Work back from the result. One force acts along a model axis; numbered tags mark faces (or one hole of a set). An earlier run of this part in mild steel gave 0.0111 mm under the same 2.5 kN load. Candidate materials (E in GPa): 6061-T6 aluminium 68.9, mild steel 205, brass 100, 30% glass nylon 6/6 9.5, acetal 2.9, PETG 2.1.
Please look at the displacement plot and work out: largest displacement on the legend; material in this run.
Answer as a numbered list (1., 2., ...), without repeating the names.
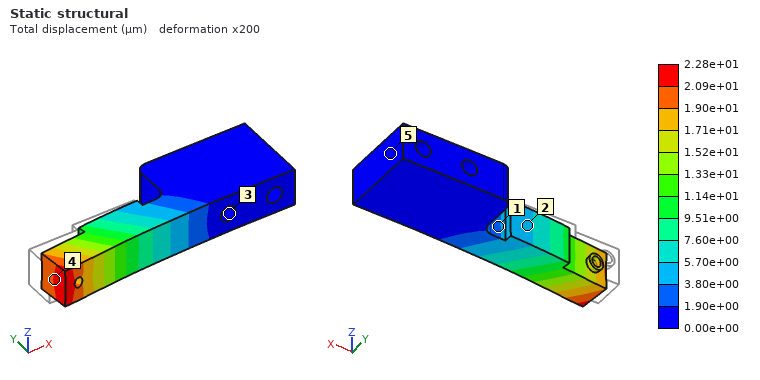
1. 2.28e+01 µm
2. brass
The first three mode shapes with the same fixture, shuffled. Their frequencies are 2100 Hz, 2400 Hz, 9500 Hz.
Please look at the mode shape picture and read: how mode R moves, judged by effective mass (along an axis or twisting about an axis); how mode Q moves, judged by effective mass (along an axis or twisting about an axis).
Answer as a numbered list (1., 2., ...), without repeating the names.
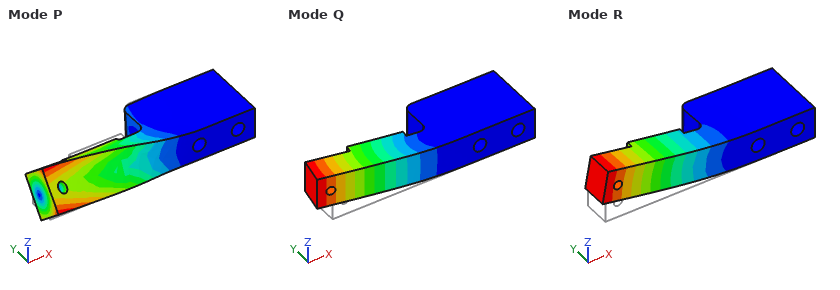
1. along Z
2. along Y
